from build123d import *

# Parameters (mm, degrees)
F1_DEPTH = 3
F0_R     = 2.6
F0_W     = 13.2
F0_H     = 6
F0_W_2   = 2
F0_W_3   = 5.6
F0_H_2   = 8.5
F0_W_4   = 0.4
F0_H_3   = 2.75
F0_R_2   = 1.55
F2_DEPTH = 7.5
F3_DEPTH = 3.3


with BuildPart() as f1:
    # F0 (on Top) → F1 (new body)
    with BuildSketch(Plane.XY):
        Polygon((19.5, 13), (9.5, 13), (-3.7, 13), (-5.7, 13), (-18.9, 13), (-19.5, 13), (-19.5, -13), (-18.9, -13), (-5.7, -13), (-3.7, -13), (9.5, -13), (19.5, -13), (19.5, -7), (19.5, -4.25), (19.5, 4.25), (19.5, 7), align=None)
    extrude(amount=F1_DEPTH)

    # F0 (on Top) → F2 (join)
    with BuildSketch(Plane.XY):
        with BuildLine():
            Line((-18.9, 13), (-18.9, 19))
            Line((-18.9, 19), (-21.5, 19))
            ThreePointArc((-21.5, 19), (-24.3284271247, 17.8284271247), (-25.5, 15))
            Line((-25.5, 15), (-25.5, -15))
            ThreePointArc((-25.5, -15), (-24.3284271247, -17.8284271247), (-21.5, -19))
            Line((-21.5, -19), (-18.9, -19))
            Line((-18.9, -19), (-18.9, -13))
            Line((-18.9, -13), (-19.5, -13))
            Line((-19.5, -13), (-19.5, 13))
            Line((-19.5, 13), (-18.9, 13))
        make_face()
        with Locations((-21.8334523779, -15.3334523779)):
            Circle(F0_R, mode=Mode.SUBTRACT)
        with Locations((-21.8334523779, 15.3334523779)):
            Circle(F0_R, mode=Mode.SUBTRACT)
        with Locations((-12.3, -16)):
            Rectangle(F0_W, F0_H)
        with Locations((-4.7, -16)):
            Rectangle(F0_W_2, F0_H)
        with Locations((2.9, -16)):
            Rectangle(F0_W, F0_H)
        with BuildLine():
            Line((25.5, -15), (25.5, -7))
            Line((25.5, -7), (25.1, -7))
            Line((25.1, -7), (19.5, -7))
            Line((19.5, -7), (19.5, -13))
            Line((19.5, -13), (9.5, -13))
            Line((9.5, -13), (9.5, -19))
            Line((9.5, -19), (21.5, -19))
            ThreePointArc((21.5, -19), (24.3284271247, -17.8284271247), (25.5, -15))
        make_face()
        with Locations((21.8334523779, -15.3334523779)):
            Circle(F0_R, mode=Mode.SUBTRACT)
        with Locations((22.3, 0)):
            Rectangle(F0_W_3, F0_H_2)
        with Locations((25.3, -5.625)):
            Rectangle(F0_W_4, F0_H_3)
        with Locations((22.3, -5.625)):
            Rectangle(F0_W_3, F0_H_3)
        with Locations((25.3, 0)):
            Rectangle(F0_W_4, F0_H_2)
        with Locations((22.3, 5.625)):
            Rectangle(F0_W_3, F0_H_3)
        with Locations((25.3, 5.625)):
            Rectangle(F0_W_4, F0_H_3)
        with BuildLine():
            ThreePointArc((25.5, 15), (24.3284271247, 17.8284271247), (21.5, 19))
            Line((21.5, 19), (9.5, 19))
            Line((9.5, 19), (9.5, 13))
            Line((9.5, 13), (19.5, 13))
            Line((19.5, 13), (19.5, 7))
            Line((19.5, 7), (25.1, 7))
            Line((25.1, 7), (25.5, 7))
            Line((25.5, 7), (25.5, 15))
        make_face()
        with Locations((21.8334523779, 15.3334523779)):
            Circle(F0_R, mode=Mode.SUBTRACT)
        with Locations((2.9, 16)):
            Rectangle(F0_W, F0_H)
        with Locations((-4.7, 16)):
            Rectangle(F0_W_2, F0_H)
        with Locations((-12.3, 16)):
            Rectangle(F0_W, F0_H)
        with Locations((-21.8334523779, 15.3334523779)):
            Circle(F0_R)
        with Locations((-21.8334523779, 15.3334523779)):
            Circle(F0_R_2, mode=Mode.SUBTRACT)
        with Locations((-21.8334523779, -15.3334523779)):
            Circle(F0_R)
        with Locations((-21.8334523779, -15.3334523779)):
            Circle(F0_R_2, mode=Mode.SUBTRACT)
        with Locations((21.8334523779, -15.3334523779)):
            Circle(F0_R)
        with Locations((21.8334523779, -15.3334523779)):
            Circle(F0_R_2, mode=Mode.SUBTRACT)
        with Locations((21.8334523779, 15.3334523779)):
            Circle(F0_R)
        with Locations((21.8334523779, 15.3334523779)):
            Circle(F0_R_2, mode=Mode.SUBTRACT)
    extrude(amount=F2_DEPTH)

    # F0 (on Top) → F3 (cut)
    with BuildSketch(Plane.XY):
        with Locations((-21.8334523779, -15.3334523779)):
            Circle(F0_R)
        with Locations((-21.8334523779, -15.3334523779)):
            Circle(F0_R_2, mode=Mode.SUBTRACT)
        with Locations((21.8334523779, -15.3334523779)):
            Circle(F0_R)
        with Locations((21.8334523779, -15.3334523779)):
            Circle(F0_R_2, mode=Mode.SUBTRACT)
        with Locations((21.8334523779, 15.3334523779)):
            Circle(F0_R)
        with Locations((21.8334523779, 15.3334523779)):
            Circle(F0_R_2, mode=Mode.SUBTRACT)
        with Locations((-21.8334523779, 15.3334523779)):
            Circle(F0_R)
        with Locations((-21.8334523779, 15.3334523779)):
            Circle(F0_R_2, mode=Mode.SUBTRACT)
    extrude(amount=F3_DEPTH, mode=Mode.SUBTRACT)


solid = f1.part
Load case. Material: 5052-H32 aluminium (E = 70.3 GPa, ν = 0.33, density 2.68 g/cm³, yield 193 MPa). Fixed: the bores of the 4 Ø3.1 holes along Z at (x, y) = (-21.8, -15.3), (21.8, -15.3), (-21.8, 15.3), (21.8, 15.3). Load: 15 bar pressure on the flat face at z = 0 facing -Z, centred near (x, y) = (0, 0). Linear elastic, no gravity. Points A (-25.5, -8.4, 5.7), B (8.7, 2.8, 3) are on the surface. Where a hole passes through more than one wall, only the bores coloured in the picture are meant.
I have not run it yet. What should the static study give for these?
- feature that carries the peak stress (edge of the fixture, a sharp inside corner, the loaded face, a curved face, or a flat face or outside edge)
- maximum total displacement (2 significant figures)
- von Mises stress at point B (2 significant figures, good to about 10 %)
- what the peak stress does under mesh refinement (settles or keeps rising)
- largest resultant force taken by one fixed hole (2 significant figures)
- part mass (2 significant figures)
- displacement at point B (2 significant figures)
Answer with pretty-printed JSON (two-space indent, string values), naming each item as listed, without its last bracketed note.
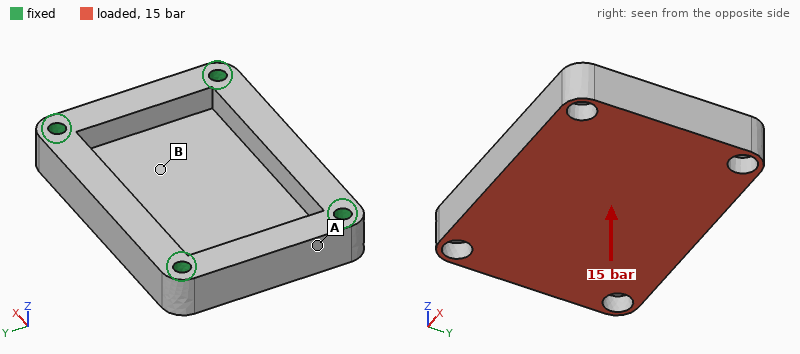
{
  "feature that carries the peak stress": "edge of the fixture",
  "maximum total displacement": "43 µm",
  "von Mises stress at point B": "23 MPa",
  "what the peak stress does under mesh refinement": "keeps rising",
  "largest resultant force taken by one fixed hole": "950 N",
  "part mass": "25 g",
  "displacement at point B": "34 µm"
}
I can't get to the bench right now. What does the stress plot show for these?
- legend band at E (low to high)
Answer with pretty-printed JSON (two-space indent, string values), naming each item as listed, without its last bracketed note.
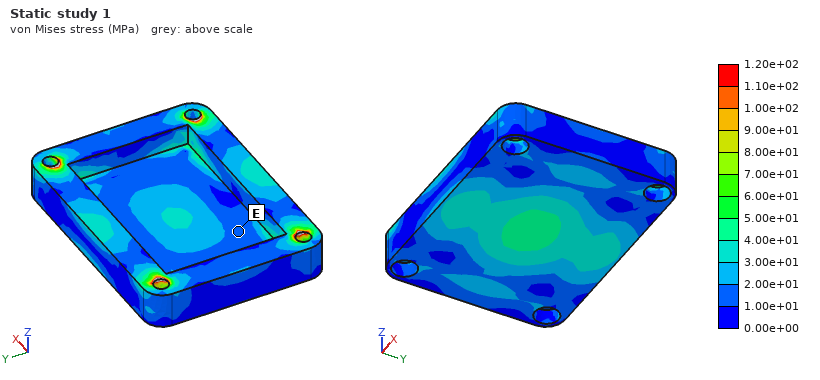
{
  "legend band at E": "1.00e+01 to 2.00e+01 MPa"
}
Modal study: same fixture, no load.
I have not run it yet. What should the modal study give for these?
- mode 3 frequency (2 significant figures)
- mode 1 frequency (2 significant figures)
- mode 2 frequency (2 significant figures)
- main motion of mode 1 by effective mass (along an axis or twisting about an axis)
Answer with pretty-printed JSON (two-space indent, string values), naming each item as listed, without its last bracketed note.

{
  "mode 3 frequency": "20 kHz",
  "mode 1 frequency": "12 kHz",
  "mode 2 frequency": "15 kHz",
  "main motion of mode 1 by effective mass": "along Z"
}
